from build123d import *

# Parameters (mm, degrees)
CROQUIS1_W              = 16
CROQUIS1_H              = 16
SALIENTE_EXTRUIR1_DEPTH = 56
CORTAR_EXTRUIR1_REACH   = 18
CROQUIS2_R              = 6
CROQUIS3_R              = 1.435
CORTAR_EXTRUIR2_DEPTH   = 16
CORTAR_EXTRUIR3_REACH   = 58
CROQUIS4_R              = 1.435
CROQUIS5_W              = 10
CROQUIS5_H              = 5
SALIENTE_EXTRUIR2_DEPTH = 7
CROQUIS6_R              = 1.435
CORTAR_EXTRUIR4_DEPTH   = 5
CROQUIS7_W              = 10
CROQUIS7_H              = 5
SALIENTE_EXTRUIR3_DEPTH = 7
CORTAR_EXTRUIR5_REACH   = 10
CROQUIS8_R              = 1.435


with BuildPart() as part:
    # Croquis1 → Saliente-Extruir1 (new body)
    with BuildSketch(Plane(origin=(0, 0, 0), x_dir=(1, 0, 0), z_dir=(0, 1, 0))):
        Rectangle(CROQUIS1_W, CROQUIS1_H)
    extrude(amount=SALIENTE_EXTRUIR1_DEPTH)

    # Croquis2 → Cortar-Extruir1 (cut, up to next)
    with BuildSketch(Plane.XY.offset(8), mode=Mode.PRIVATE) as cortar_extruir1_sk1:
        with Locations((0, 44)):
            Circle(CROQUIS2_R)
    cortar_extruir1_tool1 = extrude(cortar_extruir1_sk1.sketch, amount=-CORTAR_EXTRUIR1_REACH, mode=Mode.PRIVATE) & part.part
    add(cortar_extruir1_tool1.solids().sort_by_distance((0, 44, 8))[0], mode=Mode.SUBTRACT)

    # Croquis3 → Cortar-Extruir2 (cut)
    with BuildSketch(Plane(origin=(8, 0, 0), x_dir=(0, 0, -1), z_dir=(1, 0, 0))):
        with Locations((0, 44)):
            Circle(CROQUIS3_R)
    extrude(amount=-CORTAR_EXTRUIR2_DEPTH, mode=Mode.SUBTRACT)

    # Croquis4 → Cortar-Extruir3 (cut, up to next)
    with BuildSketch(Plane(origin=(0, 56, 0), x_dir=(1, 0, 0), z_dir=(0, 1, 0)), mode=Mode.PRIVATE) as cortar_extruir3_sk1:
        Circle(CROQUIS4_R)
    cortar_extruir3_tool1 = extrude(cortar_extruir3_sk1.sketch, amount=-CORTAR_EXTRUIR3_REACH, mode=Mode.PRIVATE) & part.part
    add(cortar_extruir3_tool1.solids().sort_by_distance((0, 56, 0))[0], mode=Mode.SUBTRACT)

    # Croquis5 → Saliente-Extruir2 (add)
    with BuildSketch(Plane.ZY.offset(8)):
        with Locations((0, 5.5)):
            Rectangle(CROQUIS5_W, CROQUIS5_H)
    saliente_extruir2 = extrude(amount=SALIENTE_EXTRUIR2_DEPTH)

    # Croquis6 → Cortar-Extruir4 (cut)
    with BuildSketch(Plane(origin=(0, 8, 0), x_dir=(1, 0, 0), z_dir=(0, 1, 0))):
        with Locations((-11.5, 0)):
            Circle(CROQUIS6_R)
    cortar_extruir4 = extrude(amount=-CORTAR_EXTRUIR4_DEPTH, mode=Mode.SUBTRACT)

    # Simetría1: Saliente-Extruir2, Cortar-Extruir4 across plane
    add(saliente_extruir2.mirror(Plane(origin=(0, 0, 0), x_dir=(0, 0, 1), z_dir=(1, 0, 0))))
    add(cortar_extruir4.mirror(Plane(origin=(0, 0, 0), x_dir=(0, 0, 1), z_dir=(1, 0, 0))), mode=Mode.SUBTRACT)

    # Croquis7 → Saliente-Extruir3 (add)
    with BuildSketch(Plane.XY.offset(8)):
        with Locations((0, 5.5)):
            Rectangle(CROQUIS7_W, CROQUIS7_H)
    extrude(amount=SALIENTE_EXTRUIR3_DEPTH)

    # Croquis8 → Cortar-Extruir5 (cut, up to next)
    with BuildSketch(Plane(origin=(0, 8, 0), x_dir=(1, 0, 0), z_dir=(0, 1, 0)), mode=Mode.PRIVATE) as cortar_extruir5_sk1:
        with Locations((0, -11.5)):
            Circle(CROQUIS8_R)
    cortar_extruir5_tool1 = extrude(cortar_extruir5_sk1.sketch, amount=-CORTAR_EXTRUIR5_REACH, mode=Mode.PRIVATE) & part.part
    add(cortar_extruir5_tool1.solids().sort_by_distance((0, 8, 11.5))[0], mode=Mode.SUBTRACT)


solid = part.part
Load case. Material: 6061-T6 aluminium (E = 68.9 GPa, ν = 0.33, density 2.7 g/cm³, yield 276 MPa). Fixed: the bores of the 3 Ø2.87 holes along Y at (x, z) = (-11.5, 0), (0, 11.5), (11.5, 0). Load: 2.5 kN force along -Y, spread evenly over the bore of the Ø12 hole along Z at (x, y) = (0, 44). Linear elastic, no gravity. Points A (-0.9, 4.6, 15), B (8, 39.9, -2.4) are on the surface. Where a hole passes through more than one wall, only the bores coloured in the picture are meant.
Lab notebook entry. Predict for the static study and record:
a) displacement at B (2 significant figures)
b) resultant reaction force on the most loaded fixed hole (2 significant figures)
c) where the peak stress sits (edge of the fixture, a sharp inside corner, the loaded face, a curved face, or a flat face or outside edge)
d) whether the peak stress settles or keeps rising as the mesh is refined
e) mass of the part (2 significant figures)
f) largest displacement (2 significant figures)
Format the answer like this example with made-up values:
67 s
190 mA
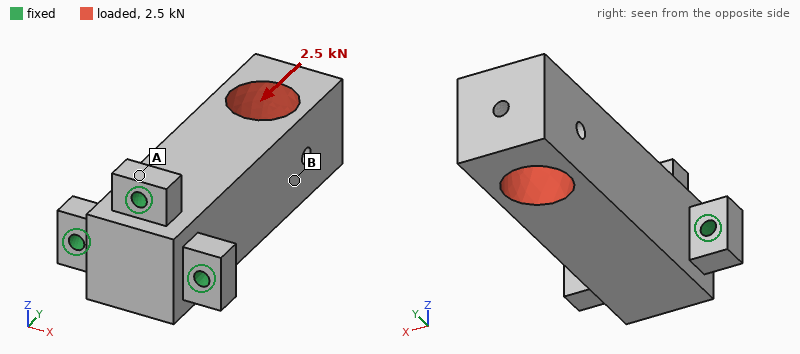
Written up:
24 µm
1.1 kN
edge of the fixture
keeps rising
36 g
35 µm
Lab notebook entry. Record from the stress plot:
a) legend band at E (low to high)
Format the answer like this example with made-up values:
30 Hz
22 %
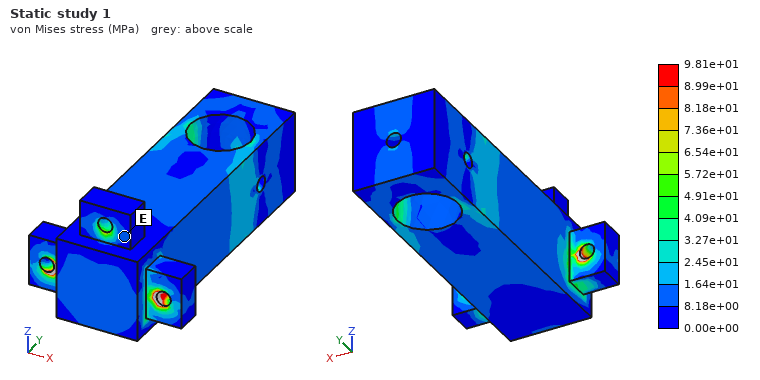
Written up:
8.18e+00 to 1.64e+01 MPa
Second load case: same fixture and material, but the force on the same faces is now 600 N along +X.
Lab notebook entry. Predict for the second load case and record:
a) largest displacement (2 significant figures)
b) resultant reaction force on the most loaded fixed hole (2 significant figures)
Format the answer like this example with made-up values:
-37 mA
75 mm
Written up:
85 µm
1.1 kN
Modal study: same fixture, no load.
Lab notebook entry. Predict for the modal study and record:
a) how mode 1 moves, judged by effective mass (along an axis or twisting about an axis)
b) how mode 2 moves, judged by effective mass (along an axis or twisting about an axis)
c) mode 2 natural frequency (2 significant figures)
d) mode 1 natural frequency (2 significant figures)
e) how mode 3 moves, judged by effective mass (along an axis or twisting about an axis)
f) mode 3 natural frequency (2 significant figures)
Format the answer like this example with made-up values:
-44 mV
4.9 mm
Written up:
along Z
along X
4200 Hz
3300 Hz
twisting about Y
14 kHz
